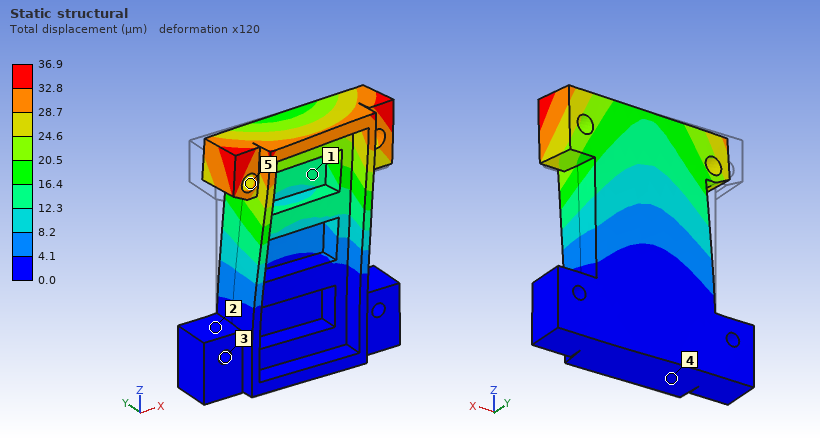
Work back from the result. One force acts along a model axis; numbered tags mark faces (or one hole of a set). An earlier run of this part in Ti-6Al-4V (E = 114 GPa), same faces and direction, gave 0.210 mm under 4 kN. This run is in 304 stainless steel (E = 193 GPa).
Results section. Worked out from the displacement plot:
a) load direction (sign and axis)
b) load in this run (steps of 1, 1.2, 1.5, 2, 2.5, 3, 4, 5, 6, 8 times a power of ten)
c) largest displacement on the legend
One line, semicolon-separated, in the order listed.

+X; 1.2 kN; 36.9 µm
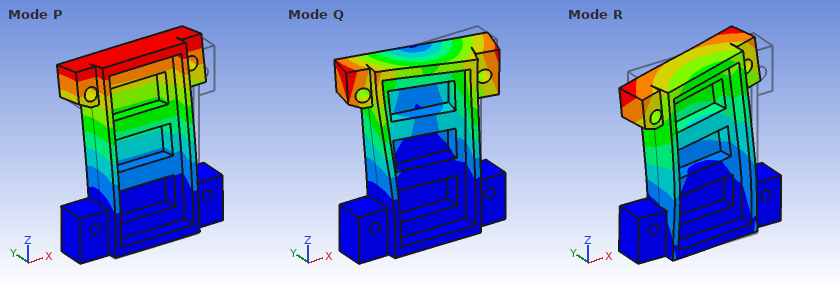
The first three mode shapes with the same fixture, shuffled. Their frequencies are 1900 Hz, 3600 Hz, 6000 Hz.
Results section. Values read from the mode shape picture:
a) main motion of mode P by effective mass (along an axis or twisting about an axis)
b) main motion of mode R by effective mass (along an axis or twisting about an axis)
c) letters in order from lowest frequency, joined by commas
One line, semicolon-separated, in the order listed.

along Y; along X; P, Q, R
